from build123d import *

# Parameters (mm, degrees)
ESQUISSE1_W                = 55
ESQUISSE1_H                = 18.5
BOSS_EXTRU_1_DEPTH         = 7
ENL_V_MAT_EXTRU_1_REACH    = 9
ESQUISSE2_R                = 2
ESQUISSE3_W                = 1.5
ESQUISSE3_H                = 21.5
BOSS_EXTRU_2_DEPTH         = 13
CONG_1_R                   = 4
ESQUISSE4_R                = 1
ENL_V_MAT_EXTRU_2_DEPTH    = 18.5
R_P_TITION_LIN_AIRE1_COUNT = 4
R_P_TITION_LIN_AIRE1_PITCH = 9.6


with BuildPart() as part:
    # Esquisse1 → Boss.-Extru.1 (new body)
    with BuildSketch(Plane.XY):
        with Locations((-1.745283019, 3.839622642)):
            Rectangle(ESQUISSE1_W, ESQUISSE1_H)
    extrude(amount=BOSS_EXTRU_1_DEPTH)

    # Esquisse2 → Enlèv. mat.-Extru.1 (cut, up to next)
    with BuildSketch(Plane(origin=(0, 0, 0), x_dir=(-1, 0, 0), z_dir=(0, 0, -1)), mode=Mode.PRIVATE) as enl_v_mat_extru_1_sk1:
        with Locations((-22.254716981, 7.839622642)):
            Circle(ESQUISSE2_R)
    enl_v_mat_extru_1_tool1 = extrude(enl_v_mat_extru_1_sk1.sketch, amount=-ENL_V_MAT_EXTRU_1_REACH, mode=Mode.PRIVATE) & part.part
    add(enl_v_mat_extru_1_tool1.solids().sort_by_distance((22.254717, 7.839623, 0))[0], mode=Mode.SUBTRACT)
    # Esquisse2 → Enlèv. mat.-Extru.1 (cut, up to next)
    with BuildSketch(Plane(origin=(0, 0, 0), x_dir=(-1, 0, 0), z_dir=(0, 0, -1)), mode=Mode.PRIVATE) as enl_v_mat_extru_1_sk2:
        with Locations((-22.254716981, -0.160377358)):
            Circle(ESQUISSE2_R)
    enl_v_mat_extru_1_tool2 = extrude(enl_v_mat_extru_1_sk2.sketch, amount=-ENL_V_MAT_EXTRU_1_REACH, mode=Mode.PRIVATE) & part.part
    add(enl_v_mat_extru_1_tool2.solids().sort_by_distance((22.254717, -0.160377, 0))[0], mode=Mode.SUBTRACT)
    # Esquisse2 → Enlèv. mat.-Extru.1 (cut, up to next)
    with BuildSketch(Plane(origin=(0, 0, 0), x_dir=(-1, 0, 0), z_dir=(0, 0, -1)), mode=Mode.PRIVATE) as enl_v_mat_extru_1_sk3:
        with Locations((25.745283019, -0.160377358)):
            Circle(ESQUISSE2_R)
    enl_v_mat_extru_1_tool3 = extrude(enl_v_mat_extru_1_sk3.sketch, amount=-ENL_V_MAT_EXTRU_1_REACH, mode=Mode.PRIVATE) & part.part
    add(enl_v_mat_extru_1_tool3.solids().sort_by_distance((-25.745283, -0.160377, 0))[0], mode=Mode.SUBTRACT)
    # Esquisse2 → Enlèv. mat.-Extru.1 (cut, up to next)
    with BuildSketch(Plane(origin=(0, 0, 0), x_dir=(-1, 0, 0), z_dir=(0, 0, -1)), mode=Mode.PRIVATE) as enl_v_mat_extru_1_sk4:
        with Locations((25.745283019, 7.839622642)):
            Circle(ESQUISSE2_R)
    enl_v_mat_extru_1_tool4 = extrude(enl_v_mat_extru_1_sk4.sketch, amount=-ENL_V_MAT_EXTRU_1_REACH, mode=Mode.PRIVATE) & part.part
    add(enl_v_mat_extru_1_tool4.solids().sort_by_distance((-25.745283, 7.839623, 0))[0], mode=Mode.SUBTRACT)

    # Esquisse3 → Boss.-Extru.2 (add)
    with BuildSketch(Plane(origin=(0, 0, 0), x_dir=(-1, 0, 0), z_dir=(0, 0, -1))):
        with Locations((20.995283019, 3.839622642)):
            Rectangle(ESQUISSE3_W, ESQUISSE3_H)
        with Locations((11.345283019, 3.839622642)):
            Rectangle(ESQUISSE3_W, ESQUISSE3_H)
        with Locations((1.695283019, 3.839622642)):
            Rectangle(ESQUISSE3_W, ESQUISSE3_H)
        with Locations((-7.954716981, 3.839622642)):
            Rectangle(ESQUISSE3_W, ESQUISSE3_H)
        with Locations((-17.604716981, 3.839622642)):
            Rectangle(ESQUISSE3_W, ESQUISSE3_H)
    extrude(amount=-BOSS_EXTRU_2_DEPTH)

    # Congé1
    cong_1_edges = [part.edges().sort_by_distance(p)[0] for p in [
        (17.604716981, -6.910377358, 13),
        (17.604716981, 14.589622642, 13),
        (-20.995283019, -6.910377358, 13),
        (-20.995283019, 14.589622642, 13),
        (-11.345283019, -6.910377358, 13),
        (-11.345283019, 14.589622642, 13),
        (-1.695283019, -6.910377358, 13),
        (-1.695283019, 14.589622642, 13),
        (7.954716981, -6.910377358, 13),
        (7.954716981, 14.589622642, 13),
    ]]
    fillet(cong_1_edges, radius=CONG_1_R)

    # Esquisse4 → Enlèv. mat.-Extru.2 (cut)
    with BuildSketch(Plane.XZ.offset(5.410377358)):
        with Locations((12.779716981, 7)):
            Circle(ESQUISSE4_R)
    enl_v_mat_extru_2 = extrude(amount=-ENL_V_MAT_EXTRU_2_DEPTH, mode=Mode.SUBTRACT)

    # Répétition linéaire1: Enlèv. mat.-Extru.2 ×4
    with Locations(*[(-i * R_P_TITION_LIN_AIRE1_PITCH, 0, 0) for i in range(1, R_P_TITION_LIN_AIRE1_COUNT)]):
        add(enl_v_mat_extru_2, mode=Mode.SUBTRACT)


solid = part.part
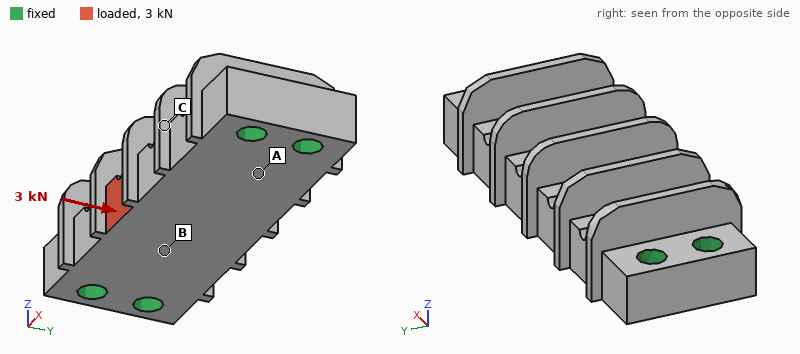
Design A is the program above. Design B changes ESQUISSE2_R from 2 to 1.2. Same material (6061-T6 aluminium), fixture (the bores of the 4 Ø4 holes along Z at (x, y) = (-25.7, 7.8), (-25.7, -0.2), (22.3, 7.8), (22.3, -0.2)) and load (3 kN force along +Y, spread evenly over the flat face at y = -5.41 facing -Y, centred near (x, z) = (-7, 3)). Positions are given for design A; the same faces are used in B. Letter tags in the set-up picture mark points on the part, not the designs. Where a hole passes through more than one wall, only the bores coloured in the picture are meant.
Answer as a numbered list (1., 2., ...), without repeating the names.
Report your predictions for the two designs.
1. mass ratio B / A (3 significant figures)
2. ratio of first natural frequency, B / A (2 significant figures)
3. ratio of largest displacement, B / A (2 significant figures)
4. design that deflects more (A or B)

1. 1.03
2. 0.91
3. 1.1
4. B
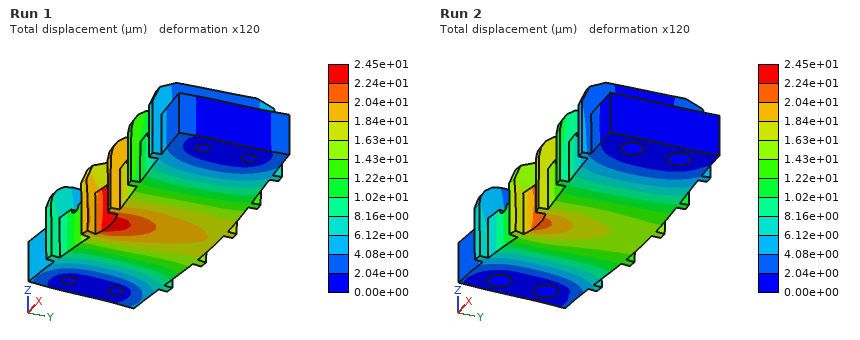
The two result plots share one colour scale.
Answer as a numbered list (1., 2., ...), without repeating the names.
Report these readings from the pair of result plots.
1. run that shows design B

1. Run 1
